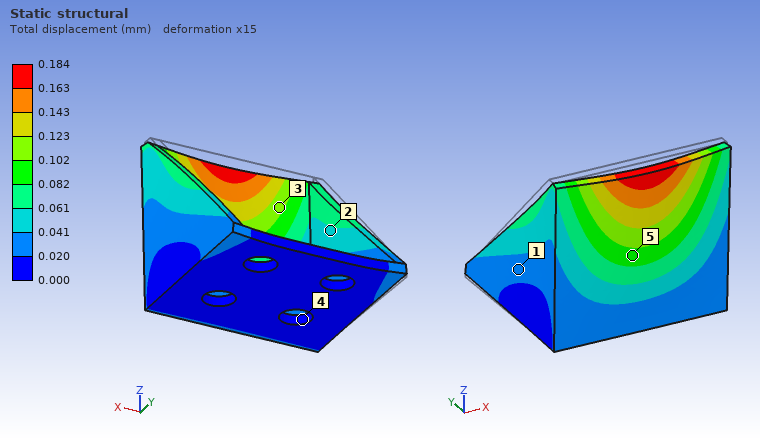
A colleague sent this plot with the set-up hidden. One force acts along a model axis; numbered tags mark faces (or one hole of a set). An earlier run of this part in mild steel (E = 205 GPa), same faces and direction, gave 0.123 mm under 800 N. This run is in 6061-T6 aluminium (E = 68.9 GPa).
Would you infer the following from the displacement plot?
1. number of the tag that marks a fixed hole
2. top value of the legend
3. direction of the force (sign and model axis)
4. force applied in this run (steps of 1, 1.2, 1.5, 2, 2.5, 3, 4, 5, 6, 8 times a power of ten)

4
0.184 mm
-Y
400 N
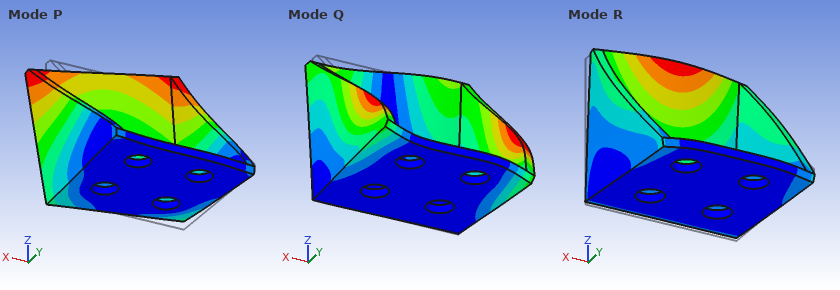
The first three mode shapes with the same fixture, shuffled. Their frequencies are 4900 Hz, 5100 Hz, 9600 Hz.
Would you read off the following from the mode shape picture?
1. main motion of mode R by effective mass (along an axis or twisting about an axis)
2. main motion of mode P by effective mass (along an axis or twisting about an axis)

along Y
along X
